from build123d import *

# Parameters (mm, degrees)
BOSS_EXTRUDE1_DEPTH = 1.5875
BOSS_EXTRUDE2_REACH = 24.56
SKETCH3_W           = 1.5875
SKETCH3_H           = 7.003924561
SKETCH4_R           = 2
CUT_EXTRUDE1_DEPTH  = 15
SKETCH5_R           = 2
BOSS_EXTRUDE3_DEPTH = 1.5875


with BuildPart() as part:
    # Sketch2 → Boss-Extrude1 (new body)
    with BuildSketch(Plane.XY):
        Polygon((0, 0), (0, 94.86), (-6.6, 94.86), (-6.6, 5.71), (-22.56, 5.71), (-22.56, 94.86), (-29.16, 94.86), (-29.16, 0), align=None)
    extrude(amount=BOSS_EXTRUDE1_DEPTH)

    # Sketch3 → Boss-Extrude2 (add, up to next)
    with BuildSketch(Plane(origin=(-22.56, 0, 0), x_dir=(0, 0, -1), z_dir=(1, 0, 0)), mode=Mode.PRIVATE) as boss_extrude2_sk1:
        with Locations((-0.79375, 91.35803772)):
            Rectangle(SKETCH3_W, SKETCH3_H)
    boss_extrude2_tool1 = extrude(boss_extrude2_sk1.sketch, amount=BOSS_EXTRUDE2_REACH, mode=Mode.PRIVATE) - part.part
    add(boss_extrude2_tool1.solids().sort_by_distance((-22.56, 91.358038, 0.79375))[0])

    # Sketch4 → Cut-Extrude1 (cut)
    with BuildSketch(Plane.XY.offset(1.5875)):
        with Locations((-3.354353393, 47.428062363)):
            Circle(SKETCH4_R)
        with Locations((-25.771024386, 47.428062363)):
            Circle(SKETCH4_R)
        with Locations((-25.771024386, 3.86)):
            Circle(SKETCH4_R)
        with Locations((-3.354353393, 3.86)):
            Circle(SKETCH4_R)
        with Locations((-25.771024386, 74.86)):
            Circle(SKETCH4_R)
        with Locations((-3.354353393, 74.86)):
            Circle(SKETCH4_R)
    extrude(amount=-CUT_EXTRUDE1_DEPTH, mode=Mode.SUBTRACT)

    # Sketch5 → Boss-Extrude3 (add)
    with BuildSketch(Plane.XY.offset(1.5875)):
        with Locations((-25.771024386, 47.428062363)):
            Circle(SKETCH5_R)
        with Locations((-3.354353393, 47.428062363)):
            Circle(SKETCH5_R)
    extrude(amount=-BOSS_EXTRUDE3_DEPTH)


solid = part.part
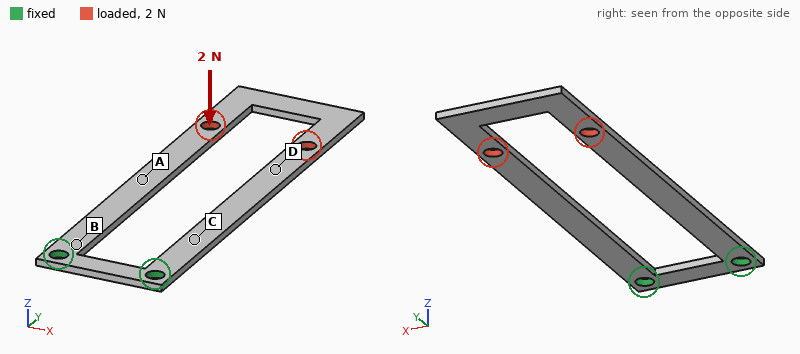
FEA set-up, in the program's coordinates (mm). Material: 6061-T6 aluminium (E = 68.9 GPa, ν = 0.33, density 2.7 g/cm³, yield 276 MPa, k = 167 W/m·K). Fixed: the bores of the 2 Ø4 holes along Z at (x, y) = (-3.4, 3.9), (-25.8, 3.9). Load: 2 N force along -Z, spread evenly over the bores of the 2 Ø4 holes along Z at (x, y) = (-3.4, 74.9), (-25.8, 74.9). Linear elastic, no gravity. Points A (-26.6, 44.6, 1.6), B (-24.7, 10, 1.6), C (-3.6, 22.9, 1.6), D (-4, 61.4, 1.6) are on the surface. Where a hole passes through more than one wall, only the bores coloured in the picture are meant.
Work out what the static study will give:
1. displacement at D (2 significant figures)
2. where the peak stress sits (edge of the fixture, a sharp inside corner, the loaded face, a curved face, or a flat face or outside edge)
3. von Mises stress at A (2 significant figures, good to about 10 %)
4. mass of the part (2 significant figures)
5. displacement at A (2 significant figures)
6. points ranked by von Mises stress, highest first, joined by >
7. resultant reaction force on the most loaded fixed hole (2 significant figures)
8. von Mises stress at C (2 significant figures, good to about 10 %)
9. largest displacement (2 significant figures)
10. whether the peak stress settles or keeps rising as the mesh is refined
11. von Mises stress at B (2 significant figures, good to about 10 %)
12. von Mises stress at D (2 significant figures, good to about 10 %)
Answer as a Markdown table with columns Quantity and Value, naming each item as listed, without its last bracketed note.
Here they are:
| Quantity | Value |
|---|---|
| displacement at D | 0.52 mm |
| where the peak stress sits | edge of the fixture |
| von Mises stress at A | 11 MPa |
| mass of the part | 6.0 g |
| displacement at A | 0.28 mm |
| points ranked by von Mises stress, highest first, joined by > | B > C > A > D |
| resultant reaction force on the most loaded fixed hole | 1.0 N |
| von Mises stress at C | 19 MPa |
| largest displacement | 1.0 mm |
| whether the peak stress settles or keeps rising as the mesh is refined | keeps rising |
| von Mises stress at B | 23 MPa |
| von Mises stress at D | 4.9 MPa |
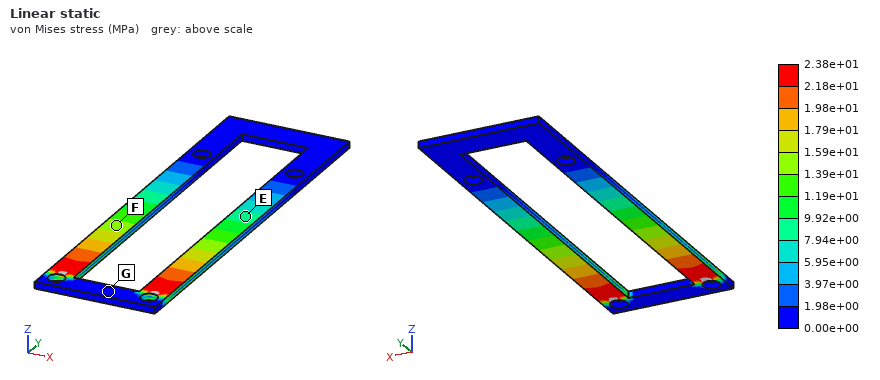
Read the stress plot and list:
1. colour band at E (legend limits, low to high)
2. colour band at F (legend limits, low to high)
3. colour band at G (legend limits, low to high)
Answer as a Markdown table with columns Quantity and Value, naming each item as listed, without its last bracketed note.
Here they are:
| Quantity | Value |
|---|---|
| colour band at E | 7.94e+00 to 9.92e+00 MPa |
| colour band at F | 1.39e+01 to 1.59e+01 MPa |
| colour band at G | 0.00e+00 to 1.98e+00 MPa |
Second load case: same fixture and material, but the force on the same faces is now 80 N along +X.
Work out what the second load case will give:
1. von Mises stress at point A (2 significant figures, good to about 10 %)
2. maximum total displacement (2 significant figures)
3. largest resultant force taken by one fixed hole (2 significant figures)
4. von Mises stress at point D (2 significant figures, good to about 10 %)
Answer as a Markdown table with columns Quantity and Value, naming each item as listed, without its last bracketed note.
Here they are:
| Quantity | Value |
|---|---|
| von Mises stress at point A | 15 MPa |
| maximum total displacement | 0.87 mm |
| largest resultant force taken by one fixed hole | 120 N |
| von Mises stress at point D | 21 MPa |
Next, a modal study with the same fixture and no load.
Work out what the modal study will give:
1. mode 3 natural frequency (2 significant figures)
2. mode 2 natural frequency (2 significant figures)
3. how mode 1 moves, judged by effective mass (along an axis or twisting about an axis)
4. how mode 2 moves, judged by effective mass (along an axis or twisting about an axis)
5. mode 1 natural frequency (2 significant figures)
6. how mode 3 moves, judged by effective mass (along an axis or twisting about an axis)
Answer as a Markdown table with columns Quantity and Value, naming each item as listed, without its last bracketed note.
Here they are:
| Quantity | Value |
|---|---|
| mode 3 natural frequency | 910 Hz |
| mode 2 natural frequency | 630 Hz |
| how mode 1 moves, judged by effective mass | along Z |
| how mode 2 moves, judged by effective mass | twisting about Y |
| mode 1 natural frequency | 140 Hz |
| how mode 3 moves, judged by effective mass | along Z |
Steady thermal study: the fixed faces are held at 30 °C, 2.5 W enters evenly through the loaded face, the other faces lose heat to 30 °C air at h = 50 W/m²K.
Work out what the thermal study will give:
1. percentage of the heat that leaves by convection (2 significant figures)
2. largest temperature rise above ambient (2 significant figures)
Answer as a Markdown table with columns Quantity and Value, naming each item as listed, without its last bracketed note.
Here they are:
| Quantity | Value |
|---|---|
| percentage of the heat that leaves by convection | 71 % |
| largest temperature rise above ambient | 21 K |
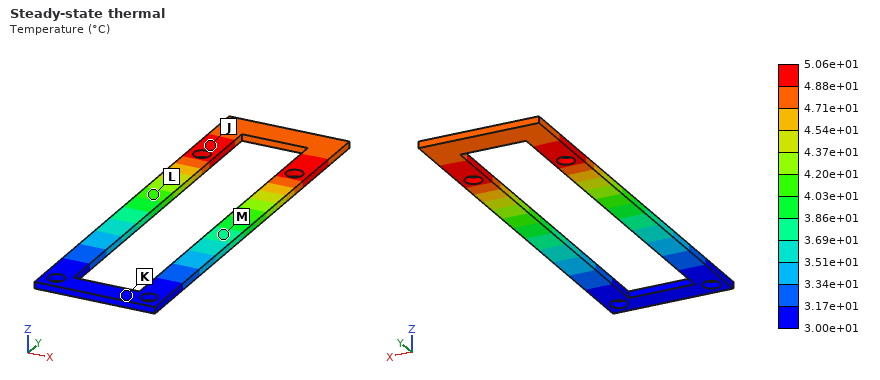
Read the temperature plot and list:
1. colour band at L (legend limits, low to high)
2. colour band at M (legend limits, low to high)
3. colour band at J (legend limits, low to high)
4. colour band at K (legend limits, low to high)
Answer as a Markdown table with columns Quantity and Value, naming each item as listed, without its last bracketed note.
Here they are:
| Quantity | Value |
|---|---|
| colour band at L | 4.03e+01 to 4.20e+01 °C |
| colour band at M | 3.69e+01 to 3.86e+01 °C |
| colour band at J | 4.88e+01 to 5.06e+01 °C |
| colour band at K | 3.00e+01 to 3.17e+01 °C |
